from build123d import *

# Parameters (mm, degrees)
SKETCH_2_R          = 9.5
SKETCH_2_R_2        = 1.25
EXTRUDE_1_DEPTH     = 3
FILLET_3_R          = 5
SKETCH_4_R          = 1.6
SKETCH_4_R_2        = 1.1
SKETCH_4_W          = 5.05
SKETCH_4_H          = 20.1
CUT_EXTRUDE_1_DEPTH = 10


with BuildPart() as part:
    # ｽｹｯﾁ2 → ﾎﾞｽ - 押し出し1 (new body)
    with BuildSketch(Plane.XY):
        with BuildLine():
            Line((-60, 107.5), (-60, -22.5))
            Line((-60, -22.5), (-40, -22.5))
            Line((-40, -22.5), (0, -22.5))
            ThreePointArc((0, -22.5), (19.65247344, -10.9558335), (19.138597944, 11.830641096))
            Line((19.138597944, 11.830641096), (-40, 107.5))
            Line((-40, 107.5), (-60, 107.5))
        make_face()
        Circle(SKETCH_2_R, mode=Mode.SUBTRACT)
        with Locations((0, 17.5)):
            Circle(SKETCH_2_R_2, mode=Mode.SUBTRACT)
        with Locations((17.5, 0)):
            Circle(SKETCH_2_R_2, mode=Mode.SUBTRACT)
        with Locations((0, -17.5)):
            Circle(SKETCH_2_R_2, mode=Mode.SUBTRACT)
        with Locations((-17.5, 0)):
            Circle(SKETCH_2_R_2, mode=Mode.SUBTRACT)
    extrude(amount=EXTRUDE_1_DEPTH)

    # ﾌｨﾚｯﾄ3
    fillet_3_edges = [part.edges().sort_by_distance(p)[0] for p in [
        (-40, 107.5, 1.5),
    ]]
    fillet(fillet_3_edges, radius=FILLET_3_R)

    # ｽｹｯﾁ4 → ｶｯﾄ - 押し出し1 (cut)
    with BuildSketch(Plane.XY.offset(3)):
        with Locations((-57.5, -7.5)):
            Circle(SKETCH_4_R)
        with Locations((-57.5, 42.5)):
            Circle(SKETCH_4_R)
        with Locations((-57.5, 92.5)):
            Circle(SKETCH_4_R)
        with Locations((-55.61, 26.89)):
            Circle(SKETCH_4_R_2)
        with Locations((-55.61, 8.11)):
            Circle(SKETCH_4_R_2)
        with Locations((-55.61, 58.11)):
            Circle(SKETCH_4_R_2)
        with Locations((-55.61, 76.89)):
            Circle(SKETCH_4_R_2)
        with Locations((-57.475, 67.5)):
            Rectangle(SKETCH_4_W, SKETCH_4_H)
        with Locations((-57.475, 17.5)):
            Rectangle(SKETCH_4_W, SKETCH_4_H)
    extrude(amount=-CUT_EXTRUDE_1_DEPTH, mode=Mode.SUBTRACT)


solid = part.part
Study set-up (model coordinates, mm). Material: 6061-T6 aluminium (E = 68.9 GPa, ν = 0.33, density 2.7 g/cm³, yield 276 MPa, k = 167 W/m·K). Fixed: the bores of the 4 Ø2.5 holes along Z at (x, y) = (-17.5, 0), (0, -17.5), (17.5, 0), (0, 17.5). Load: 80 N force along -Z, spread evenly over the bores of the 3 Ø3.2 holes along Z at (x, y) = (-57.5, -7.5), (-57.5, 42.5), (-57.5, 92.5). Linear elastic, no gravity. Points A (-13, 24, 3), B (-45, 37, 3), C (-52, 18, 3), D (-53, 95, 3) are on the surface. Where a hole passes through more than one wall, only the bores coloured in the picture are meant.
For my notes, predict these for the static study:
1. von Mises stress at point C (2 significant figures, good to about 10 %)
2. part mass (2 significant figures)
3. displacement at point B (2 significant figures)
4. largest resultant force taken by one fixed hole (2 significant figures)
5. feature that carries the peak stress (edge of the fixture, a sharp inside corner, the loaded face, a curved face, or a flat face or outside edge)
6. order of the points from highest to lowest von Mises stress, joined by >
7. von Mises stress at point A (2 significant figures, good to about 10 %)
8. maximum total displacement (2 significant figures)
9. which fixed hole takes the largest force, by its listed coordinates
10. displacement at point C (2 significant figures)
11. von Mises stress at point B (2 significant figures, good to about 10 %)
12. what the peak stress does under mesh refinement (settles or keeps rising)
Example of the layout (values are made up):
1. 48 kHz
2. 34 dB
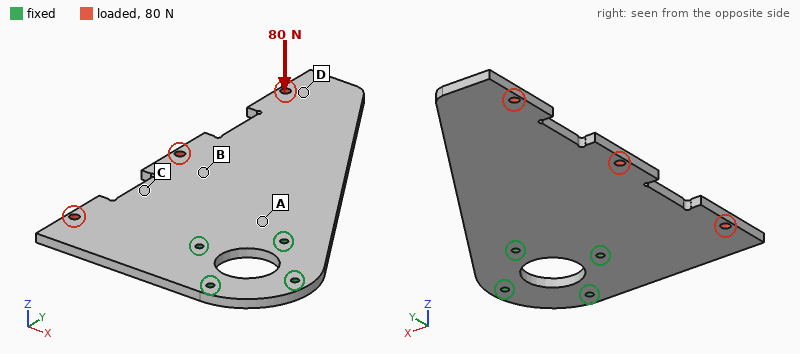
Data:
1. 26 MPa
2. 56 g
3. 0.39 mm
4. 110 N
5. edge of the fixture
6. A > C > B > D
7. 34 MPa
8. 1.5 mm
9. (-17.5, 0)
10. 0.25 mm
11. 18 MPa
12. keeps rising
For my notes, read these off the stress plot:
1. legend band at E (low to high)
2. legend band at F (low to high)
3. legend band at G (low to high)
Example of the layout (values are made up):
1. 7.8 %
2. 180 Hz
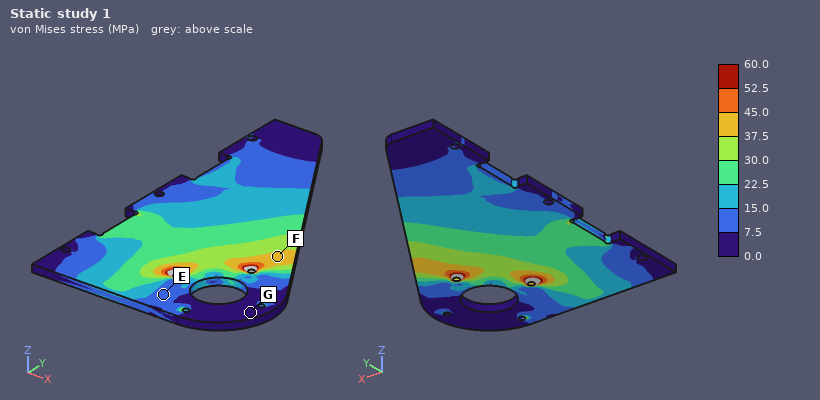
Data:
1. 7.5 to 15.0 MPa
2. 37.5 to 45.0 MPa
3. 0.0 to 7.5 MPa
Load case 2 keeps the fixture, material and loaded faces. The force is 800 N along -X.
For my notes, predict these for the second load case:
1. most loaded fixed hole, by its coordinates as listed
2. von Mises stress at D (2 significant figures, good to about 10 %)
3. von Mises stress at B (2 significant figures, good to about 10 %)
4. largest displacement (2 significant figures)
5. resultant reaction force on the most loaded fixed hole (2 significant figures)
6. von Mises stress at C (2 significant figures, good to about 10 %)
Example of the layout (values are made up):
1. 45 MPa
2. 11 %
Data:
1. (0, 17.5)
2. 8.0 MPa
3. 9.3 MPa
4. 64 µm
5. 880 N
6. 8.6 MPa
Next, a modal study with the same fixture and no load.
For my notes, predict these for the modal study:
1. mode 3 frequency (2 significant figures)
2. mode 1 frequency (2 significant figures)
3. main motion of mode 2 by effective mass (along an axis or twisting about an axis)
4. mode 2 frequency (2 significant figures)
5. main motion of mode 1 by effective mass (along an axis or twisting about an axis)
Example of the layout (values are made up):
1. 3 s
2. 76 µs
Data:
1. 1600 Hz
2. 290 Hz
3. along Z
4. 1100 Hz
5. along Z
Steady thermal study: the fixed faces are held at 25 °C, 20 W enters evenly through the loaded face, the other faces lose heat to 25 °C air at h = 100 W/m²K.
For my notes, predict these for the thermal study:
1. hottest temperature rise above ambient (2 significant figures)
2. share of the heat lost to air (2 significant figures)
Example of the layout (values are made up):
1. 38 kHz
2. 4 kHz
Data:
1. 26 K
2. 62 %
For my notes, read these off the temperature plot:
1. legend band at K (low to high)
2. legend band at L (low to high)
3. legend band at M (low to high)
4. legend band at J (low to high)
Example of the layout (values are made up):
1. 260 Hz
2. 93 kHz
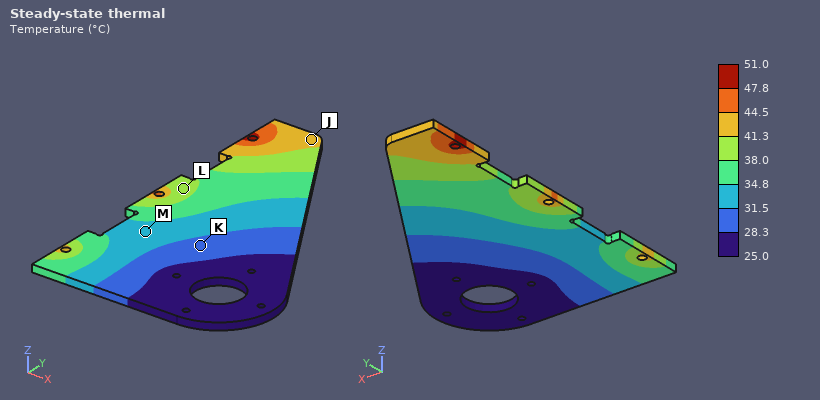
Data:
1. 28.3 to 31.5 °C
2. 38.0 to 41.3 °C
3. 31.5 to 34.8 °C
4. 41.3 to 44.5 °C
